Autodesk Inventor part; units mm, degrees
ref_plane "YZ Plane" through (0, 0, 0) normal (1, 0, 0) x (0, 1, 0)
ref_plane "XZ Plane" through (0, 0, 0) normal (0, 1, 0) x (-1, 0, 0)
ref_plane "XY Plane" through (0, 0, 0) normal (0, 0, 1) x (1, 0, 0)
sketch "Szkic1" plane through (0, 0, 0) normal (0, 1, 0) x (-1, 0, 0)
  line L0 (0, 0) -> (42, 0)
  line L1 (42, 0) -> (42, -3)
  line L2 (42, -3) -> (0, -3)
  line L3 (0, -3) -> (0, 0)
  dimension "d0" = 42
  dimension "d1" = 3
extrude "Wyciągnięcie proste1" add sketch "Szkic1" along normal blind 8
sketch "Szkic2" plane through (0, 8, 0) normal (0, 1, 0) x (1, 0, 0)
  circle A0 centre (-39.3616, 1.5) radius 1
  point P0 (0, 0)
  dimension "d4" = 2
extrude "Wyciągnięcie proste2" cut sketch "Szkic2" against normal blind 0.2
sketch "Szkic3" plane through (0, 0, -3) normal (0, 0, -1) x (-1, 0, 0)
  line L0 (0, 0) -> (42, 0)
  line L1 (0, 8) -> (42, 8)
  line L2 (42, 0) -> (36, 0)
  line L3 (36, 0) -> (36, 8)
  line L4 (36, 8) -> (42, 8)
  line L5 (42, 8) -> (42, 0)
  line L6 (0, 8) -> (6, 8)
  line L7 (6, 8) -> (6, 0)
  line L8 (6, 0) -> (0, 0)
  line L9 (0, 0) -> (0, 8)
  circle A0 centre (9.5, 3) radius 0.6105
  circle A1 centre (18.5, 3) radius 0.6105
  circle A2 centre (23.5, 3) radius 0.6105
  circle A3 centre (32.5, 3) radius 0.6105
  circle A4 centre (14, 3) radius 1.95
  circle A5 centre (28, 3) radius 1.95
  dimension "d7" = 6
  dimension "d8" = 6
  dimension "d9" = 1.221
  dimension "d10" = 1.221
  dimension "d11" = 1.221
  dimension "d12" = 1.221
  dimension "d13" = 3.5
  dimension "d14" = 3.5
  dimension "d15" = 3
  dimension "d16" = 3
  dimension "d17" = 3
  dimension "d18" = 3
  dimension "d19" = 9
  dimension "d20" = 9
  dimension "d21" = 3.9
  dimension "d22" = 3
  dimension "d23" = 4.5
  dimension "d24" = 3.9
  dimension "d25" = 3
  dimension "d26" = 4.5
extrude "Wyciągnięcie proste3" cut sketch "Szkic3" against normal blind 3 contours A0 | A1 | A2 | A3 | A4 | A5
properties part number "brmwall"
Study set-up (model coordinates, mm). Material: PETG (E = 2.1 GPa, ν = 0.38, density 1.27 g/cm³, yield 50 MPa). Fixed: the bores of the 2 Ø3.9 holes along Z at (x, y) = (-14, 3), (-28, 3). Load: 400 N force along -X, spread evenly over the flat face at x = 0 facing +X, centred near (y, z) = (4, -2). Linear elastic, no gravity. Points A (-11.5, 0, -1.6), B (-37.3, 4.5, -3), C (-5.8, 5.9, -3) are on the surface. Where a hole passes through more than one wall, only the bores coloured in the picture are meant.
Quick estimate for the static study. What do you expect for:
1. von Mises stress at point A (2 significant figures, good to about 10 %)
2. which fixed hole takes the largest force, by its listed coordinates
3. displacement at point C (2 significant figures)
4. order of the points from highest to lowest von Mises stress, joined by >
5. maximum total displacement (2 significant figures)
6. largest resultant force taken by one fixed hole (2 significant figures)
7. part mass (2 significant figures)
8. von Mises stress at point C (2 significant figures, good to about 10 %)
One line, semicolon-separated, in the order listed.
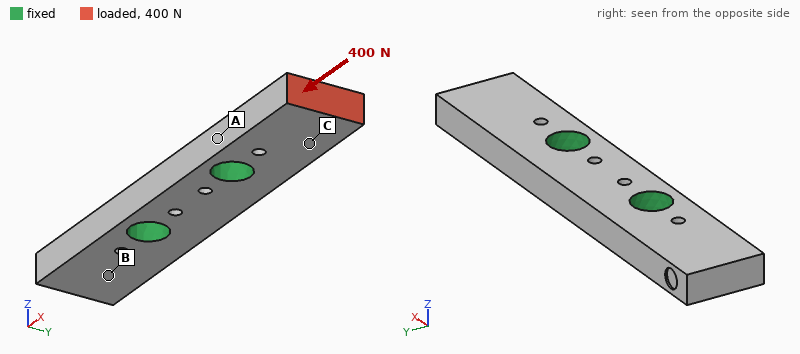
9.0 MPa; (-14, 3); 0.082 mm; C > A > B; 0.14 mm; 380 N; 1.2 g; 17 MPa
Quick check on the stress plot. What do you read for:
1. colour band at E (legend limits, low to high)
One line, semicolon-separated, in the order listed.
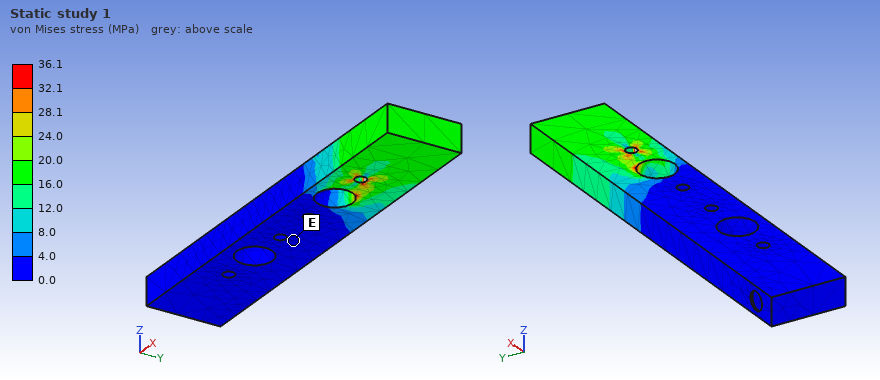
0.0 to 4.0 MPa
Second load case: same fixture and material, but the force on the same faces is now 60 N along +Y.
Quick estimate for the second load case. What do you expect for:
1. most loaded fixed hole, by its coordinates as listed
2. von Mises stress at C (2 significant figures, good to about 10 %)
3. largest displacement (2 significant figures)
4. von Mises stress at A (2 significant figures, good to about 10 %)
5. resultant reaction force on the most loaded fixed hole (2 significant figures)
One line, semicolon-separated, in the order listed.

(-14, 3); 7.1 MPa; 0.30 mm; 23 MPa; 77 N
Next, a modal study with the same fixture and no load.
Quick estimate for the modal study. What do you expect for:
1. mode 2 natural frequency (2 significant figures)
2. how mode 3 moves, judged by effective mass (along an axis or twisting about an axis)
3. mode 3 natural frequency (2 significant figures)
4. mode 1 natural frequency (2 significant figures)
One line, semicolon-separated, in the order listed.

3600 Hz; twisting about Z; 6600 Hz; 3600 Hz
